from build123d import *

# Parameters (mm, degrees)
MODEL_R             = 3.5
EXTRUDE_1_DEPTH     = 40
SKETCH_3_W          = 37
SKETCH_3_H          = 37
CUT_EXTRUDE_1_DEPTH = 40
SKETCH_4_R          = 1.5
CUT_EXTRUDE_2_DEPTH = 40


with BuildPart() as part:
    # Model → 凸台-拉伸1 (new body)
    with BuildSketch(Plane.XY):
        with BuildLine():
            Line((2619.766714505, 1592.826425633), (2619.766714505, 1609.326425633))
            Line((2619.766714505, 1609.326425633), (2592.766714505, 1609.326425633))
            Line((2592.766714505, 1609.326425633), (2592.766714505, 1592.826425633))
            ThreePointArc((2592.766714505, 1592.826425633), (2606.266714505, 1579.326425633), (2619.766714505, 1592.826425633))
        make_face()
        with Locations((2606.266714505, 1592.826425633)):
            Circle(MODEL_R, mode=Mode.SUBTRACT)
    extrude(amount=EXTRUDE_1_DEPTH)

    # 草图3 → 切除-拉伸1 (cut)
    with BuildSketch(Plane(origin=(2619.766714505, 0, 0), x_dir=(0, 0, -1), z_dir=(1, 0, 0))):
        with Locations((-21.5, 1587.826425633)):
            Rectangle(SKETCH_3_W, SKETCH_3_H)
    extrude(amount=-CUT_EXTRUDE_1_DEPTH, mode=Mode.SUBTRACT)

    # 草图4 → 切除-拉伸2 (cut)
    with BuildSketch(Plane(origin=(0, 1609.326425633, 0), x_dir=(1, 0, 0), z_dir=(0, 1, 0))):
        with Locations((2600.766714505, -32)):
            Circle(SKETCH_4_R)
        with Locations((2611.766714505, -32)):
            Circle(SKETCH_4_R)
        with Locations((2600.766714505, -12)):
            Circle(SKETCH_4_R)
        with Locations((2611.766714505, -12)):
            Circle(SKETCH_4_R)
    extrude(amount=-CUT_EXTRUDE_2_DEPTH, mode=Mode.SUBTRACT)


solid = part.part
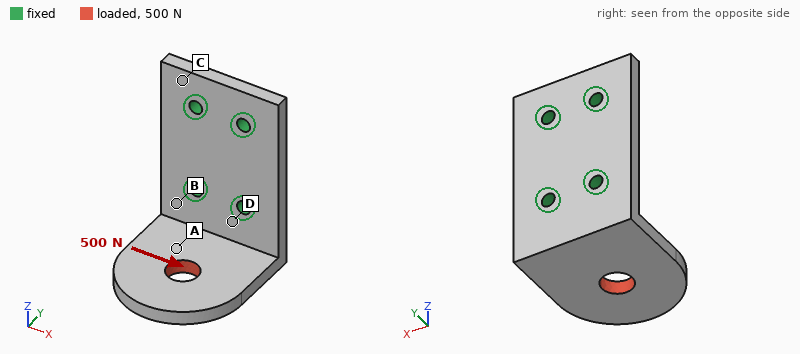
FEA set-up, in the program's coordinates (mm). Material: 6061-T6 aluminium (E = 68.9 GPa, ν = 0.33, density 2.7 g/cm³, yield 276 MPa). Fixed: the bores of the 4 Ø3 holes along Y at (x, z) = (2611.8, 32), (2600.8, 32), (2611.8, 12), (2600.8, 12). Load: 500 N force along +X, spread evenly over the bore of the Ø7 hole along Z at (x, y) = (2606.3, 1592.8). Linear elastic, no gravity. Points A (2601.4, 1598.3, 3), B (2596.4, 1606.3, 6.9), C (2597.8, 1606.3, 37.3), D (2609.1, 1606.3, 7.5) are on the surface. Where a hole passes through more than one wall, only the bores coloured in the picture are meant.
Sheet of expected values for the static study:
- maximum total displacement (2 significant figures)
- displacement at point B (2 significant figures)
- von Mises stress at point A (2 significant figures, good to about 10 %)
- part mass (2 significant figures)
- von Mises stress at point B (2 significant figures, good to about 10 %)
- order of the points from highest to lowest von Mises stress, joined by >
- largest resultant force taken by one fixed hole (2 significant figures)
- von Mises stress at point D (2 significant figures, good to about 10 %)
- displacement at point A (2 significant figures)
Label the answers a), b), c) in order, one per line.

a) 0.16 mm
b) 0.025 mm
c) 27 MPa
d) 13 g
e) 60 MPa
f) D > B > A > C
g) 630 N
h) 87 MPa
i) 0.062 mm
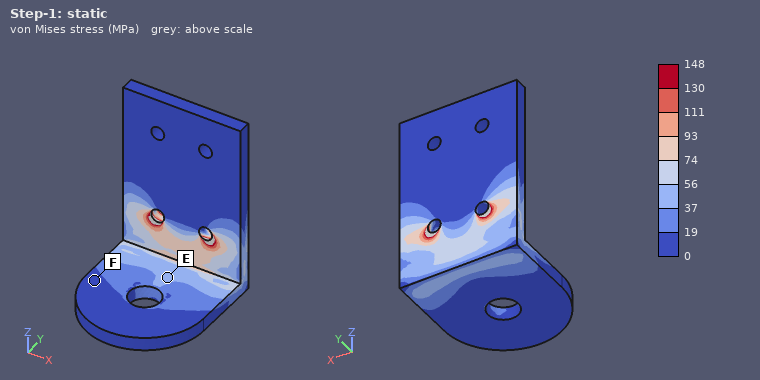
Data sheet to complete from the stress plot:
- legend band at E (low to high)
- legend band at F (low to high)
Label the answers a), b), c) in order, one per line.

a) 37 to 56 MPa
b) 0 to 19 MPa
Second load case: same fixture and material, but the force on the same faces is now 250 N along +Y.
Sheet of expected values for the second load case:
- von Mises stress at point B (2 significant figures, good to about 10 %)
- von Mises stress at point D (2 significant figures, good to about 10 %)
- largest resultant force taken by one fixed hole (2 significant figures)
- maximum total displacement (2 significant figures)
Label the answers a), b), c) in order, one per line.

a) 27 MPa
b) 35 MPa
c) 140 N
d) 93 µm
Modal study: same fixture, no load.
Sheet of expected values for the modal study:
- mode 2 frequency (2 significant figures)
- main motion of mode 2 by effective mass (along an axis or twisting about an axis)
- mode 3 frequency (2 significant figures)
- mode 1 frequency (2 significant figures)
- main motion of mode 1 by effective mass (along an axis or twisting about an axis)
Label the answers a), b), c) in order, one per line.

a) 4700 Hz
b) along X
c) 8800 Hz
d) 2300 Hz
e) along Z
